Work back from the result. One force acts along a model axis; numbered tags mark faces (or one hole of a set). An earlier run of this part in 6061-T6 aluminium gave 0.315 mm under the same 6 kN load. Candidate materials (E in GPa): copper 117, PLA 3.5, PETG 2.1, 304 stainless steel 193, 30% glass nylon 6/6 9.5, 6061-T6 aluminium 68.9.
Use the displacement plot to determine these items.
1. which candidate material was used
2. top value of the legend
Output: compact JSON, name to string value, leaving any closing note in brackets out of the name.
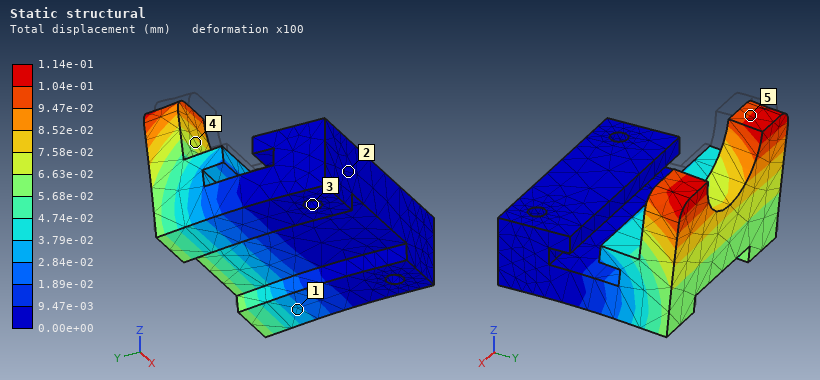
{"which candidate material was used": "304 stainless steel", "top value of the legend": "1.14e-01 mm"}
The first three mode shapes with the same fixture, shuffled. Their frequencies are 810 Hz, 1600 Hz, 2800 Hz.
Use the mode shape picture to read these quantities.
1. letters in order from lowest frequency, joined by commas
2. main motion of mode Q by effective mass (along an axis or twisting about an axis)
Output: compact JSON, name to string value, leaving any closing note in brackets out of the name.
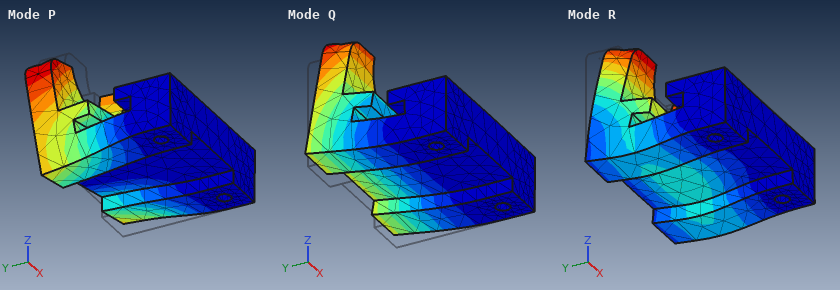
{"letters in order from lowest frequency, joined by commas": "Q, P, R", "main motion of mode Q by effective mass": "along Z"}
